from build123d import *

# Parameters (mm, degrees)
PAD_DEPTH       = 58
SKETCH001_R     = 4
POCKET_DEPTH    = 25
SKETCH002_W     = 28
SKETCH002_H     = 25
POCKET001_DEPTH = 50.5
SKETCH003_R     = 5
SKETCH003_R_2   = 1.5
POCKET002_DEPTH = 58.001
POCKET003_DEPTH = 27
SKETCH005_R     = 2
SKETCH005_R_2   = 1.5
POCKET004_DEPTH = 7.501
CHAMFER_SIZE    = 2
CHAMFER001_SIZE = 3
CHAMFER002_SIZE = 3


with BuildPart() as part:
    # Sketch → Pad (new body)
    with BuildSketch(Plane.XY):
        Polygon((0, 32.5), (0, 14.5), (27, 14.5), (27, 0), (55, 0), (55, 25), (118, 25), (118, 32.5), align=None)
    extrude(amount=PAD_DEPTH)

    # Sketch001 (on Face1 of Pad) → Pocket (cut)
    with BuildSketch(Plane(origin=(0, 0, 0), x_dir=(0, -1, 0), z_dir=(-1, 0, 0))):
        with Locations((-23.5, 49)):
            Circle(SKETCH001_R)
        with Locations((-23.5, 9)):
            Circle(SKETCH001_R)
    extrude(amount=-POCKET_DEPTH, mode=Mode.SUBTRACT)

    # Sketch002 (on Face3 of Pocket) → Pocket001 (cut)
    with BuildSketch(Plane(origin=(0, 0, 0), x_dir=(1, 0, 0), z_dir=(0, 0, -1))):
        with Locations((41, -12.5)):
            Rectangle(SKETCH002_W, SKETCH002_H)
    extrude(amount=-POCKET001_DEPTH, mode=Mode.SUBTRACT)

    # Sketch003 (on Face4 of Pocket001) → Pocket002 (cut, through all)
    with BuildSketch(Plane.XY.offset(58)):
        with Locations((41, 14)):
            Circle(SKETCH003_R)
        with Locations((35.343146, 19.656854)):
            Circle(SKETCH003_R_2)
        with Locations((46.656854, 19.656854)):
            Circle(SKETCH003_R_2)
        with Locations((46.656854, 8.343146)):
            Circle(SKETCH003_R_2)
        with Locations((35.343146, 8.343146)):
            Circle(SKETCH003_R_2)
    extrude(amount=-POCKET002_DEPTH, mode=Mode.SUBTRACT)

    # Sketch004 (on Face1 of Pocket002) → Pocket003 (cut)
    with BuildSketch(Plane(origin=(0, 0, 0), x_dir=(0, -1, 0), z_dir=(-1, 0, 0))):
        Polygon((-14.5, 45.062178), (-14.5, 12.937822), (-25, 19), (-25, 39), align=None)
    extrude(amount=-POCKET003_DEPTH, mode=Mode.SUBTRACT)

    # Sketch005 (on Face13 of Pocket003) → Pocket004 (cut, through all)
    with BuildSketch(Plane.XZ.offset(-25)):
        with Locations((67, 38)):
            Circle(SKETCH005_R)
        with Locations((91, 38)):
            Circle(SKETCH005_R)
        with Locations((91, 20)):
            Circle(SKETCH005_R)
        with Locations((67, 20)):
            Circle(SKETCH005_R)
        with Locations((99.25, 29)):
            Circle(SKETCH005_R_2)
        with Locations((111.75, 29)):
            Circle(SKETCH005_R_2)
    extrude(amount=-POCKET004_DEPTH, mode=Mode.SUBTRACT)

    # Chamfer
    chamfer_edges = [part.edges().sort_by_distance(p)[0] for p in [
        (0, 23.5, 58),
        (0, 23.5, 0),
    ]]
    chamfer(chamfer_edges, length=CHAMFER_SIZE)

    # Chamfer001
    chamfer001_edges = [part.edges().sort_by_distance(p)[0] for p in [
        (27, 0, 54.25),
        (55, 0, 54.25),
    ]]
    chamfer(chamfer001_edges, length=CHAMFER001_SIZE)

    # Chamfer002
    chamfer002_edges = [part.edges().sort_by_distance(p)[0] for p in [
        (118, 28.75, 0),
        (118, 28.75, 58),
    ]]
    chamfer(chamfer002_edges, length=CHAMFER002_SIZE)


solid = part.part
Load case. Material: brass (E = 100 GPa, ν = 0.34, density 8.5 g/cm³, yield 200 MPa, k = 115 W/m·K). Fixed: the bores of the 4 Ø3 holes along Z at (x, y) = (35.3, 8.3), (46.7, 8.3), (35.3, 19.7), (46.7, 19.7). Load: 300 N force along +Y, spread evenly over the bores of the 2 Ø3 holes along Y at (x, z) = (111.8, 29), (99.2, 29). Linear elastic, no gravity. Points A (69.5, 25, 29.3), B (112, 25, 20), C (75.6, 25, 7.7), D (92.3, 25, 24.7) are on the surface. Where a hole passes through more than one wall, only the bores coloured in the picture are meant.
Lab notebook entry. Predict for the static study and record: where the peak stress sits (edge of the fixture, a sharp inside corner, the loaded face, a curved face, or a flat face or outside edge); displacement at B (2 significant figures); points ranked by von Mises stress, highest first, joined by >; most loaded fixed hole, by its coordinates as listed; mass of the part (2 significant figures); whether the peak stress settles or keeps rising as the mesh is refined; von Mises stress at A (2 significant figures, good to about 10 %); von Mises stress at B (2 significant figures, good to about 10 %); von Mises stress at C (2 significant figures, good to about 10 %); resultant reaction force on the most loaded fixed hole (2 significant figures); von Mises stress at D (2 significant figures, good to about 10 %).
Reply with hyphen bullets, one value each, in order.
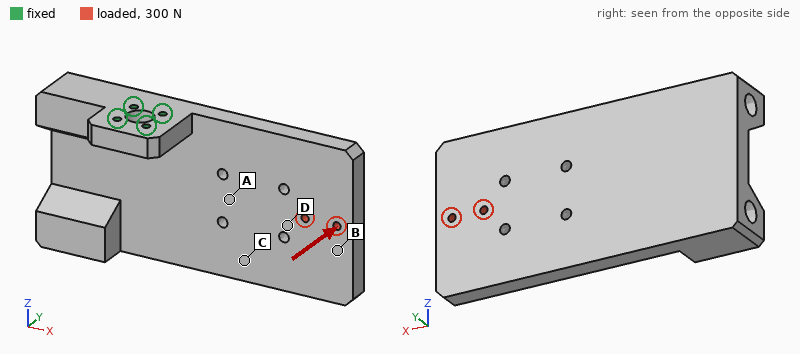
- edge of the fixture
- 0.22 mm
- A > C > D > B
- (46.7, 19.7)
- 520 g
- keeps rising
- 21 MPa
- 4.7 MPa
- 14 MPa
- 830 N
- 9.2 MPa
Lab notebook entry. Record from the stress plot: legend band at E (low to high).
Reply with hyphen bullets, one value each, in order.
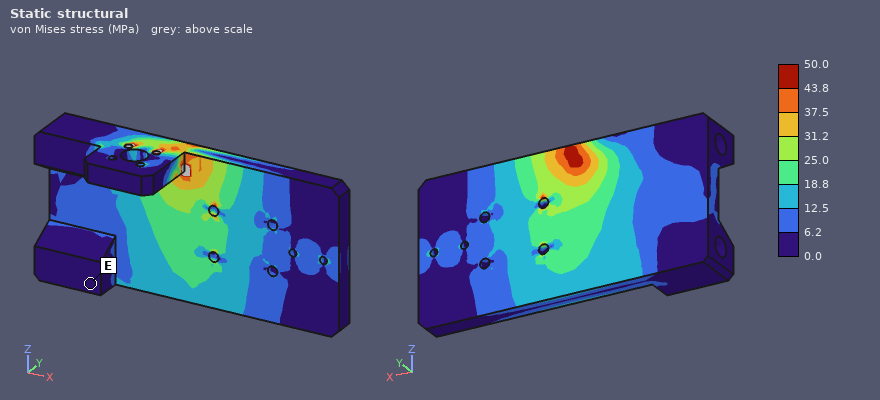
- 0.0 to 6.2 MPa
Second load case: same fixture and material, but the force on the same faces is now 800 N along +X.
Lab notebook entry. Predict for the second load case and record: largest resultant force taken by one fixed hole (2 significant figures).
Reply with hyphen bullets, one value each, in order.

- 1.1 kN
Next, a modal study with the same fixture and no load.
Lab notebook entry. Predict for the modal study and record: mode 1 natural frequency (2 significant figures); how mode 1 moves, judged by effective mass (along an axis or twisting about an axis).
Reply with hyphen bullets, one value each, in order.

- 550 Hz
- along Y
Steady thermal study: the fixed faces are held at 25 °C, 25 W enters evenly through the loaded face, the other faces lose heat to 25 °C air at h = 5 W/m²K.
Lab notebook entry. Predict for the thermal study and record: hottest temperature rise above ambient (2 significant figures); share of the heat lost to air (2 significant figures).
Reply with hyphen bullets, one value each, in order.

- 49 K
- 8.2 %
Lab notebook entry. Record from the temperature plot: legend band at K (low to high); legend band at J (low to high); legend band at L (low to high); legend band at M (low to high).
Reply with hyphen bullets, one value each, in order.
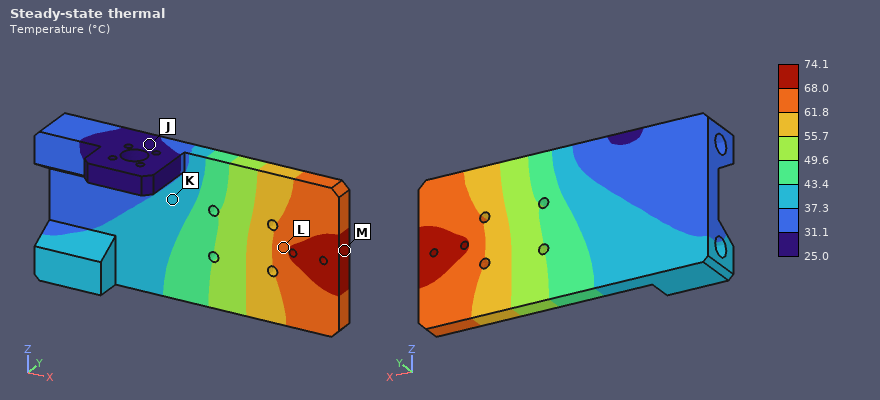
- 37.3 to 43.4 °C
- 25.0 to 31.1 °C
- 61.8 to 68.0 °C
- 68.0 to 74.1 °C
